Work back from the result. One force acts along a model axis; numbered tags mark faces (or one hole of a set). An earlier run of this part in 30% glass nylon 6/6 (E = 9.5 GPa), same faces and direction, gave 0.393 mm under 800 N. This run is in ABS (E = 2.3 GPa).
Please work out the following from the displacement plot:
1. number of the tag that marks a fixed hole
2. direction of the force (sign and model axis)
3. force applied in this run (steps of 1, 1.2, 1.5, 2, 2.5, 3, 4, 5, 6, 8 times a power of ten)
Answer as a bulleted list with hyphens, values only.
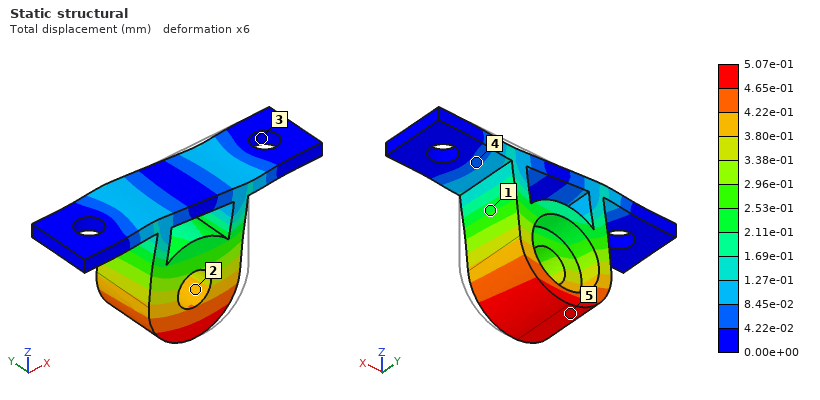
- 3
- -X
- 250 N
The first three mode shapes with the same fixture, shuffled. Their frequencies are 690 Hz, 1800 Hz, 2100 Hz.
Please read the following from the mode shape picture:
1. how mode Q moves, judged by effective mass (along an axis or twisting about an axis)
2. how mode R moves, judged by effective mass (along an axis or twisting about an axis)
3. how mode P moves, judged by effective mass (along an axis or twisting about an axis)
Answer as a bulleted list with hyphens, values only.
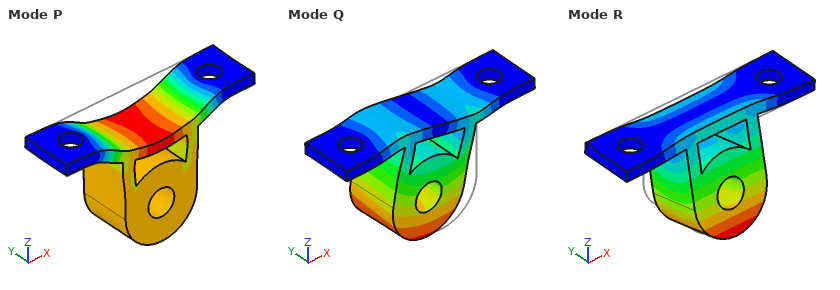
- along X
- along Y
- along Z
